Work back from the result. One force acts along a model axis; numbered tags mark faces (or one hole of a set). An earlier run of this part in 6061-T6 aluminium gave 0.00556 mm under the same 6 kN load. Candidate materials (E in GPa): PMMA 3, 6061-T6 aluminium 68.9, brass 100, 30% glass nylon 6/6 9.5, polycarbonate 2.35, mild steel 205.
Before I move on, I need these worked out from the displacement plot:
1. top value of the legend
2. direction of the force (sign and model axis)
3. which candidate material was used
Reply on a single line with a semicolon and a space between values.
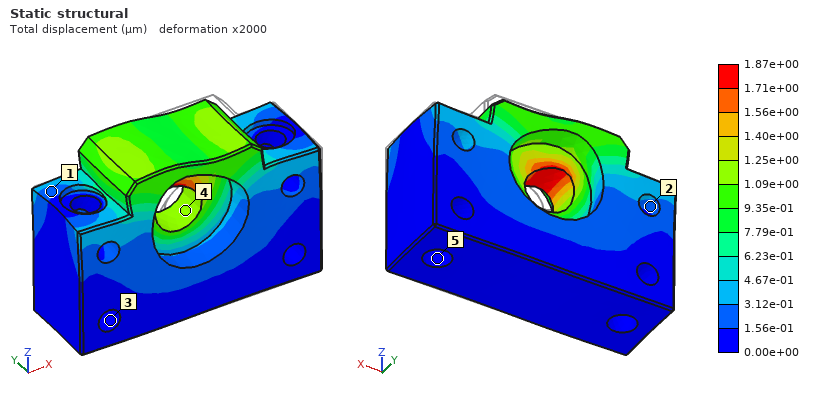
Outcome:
1.87e+00 µm; -X; mild steel
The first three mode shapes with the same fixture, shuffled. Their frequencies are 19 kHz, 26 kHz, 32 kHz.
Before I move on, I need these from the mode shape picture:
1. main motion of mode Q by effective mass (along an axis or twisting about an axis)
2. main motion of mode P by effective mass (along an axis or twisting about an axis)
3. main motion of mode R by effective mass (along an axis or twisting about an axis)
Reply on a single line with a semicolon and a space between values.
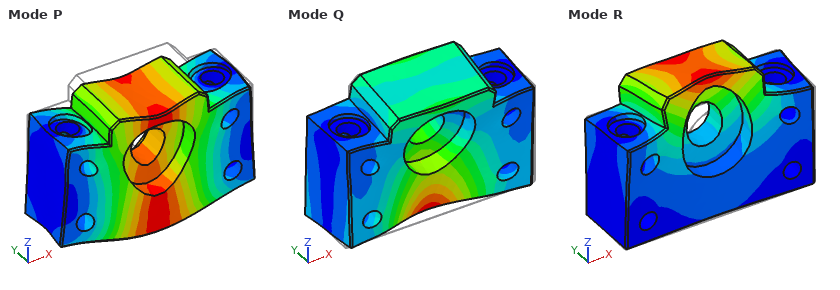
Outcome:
along Y; along Z; along Y
